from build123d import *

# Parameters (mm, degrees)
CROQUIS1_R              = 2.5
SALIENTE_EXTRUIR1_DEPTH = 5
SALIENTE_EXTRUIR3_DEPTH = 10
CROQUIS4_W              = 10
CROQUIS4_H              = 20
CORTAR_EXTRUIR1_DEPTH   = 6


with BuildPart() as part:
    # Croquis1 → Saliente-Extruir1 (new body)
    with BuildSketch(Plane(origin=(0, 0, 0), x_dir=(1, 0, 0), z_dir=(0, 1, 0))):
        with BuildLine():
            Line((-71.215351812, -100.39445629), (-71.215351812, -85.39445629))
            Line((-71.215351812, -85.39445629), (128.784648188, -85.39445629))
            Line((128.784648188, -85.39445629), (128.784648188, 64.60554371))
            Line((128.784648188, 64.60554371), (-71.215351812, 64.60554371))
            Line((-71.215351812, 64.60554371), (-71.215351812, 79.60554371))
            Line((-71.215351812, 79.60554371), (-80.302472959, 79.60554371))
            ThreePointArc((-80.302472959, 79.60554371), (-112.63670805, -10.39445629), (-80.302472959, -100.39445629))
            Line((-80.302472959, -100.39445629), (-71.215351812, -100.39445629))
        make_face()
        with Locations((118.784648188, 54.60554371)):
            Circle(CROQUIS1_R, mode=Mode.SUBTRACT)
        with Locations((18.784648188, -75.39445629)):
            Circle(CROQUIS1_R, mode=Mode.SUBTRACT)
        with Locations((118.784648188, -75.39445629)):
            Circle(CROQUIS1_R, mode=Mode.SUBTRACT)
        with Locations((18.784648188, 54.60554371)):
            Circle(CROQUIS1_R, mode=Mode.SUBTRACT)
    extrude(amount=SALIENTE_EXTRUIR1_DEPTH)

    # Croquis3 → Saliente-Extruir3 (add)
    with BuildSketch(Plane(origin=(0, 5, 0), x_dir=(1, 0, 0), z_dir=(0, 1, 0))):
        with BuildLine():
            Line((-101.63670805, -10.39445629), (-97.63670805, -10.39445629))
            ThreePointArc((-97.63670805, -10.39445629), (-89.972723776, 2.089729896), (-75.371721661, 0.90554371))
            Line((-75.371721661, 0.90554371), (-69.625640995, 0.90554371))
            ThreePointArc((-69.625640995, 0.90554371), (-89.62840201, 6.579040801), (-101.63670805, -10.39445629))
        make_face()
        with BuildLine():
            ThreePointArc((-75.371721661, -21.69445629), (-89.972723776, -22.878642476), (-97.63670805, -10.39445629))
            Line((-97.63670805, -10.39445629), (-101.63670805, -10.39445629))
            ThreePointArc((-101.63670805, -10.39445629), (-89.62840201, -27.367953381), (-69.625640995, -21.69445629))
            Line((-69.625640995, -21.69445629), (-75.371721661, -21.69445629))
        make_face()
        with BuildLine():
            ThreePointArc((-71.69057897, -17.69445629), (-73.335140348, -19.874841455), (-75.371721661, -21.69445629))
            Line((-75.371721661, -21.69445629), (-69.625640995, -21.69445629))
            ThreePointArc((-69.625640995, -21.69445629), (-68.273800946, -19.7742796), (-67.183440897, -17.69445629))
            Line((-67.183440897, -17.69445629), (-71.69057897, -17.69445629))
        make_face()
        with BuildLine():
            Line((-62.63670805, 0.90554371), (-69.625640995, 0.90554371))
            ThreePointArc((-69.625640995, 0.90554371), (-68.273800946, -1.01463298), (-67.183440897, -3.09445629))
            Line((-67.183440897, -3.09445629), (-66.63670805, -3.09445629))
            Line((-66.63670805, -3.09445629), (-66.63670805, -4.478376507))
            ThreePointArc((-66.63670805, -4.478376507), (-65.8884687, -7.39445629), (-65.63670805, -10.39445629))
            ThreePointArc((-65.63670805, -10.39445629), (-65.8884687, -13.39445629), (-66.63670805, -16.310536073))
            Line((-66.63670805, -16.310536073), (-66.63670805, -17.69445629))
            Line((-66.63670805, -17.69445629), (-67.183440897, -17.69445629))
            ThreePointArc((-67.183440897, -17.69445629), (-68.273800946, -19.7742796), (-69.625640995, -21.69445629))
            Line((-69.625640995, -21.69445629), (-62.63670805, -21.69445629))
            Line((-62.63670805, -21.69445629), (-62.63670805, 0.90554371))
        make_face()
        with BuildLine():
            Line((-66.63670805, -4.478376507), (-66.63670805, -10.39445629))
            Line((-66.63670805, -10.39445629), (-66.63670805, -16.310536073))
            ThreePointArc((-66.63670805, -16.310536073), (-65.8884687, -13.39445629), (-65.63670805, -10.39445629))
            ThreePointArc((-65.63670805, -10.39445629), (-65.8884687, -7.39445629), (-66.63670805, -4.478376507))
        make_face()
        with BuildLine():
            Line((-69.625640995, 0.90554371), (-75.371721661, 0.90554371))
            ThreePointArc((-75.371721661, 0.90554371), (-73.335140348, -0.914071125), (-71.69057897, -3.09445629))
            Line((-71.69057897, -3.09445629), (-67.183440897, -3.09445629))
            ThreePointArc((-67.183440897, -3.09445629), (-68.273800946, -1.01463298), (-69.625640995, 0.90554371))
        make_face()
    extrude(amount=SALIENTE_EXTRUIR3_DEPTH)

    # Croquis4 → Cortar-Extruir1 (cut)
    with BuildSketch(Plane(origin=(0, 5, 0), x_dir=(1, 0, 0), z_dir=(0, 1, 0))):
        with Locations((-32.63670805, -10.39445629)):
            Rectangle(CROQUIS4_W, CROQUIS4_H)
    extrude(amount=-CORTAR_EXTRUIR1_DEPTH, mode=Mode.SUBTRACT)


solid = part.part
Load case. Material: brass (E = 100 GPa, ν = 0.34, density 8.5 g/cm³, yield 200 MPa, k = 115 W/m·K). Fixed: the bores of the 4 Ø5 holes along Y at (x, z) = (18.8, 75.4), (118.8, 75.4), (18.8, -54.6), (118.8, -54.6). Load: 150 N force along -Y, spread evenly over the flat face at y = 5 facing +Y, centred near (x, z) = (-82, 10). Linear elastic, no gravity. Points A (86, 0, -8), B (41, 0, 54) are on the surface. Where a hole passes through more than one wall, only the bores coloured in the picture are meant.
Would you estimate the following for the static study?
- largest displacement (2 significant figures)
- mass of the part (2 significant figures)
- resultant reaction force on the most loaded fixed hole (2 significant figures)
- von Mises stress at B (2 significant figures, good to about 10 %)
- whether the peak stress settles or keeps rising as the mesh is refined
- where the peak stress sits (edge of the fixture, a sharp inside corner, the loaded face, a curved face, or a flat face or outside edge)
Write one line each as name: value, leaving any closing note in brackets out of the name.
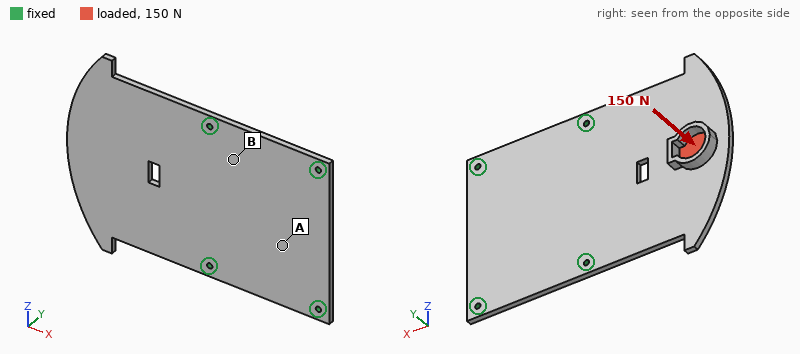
largest displacement: 0.65 mm
mass of the part: 1.5 kg
resultant reaction force on the most loaded fixed hole: 110 N
von Mises stress at B: 6.7 MPa
whether the peak stress settles or keeps rising as the mesh is refined: keeps rising
where the peak stress sits: edge of the fixture
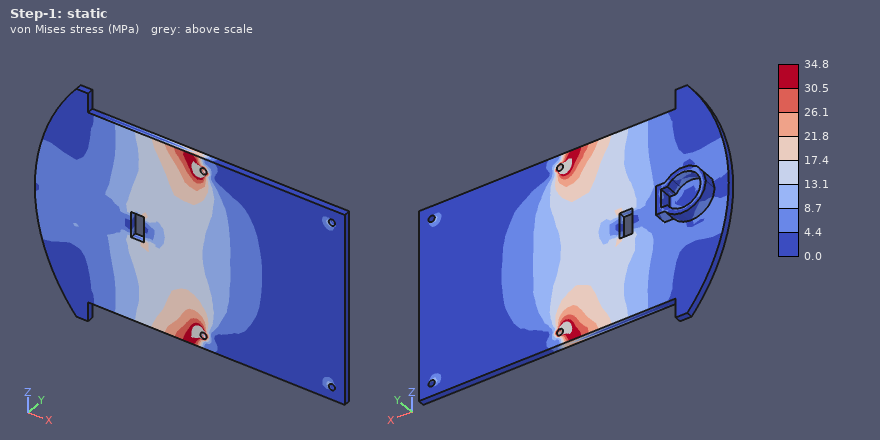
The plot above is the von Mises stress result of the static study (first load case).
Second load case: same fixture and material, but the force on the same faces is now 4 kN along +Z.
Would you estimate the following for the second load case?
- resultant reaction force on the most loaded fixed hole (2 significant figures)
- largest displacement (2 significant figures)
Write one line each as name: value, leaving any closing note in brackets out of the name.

resultant reaction force on the most loaded fixed hole: 3.4 kN
largest displacement: 0.18 mm
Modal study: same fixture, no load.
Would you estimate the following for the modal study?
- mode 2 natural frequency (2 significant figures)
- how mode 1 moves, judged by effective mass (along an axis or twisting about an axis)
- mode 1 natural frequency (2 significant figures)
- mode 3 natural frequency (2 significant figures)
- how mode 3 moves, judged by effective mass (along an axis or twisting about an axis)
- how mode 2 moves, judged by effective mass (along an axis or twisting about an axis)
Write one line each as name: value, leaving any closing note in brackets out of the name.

mode 2 natural frequency: 380 Hz
how mode 1 moves, judged by effective mass: along Y
mode 1 natural frequency: 140 Hz
mode 3 natural frequency: 790 Hz
how mode 3 moves, judged by effective mass: along Y
how mode 2 moves, judged by effective mass: twisting about X
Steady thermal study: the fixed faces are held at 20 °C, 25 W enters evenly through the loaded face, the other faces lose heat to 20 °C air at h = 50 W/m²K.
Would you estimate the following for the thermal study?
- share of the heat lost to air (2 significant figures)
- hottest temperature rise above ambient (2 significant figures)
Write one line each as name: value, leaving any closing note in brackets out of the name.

share of the heat lost to air: 78 %
hottest temperature rise above ambient: 22 K
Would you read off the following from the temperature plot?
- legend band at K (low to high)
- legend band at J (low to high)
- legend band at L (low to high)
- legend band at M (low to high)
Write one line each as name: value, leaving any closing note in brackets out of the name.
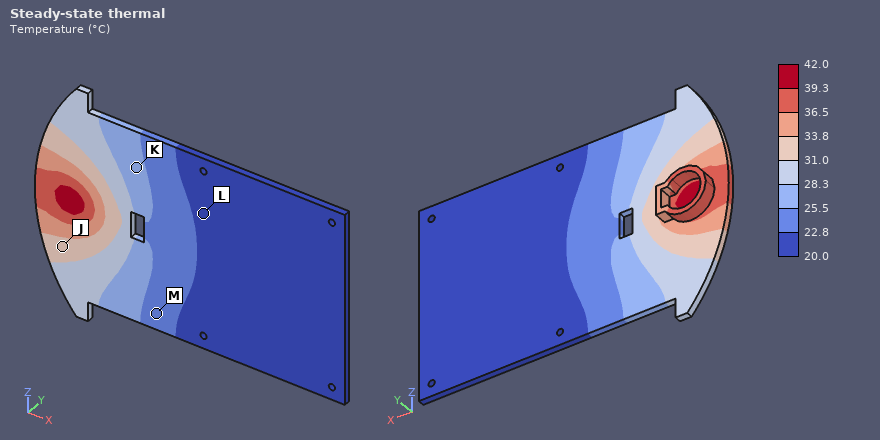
legend band at K: 25.5 to 28.3 °C
legend band at J: 31.0 to 33.8 °C
legend band at L: 20.0 to 22.8 °C
legend band at M: 22.8 to 25.5 °C
